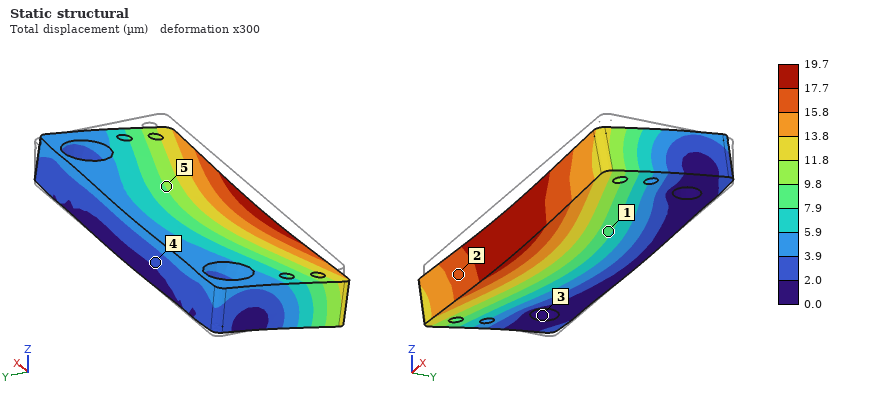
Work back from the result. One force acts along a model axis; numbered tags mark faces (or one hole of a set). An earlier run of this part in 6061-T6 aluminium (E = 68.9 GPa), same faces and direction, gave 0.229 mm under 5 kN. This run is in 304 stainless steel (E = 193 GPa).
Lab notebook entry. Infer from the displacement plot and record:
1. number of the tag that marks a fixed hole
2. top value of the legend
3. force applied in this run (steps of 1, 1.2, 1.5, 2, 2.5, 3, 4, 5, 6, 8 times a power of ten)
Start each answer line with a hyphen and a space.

- 3
- 19.7 µm
- 1.2 kN
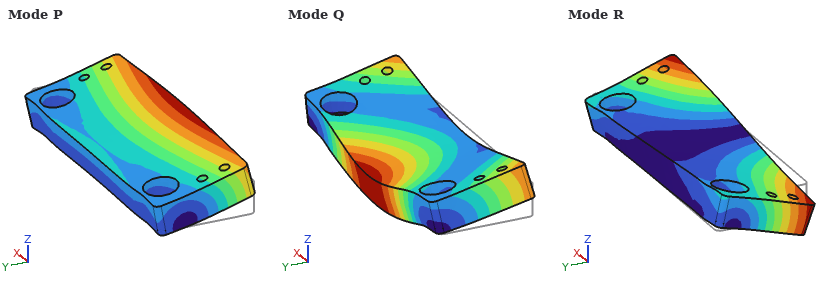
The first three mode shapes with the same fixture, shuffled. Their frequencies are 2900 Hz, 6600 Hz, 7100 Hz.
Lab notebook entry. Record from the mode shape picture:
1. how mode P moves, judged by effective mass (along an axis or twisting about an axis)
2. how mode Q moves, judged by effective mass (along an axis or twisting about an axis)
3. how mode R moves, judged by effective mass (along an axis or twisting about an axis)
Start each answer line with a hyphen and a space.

- along Z
- along Z
- twisting about Y
